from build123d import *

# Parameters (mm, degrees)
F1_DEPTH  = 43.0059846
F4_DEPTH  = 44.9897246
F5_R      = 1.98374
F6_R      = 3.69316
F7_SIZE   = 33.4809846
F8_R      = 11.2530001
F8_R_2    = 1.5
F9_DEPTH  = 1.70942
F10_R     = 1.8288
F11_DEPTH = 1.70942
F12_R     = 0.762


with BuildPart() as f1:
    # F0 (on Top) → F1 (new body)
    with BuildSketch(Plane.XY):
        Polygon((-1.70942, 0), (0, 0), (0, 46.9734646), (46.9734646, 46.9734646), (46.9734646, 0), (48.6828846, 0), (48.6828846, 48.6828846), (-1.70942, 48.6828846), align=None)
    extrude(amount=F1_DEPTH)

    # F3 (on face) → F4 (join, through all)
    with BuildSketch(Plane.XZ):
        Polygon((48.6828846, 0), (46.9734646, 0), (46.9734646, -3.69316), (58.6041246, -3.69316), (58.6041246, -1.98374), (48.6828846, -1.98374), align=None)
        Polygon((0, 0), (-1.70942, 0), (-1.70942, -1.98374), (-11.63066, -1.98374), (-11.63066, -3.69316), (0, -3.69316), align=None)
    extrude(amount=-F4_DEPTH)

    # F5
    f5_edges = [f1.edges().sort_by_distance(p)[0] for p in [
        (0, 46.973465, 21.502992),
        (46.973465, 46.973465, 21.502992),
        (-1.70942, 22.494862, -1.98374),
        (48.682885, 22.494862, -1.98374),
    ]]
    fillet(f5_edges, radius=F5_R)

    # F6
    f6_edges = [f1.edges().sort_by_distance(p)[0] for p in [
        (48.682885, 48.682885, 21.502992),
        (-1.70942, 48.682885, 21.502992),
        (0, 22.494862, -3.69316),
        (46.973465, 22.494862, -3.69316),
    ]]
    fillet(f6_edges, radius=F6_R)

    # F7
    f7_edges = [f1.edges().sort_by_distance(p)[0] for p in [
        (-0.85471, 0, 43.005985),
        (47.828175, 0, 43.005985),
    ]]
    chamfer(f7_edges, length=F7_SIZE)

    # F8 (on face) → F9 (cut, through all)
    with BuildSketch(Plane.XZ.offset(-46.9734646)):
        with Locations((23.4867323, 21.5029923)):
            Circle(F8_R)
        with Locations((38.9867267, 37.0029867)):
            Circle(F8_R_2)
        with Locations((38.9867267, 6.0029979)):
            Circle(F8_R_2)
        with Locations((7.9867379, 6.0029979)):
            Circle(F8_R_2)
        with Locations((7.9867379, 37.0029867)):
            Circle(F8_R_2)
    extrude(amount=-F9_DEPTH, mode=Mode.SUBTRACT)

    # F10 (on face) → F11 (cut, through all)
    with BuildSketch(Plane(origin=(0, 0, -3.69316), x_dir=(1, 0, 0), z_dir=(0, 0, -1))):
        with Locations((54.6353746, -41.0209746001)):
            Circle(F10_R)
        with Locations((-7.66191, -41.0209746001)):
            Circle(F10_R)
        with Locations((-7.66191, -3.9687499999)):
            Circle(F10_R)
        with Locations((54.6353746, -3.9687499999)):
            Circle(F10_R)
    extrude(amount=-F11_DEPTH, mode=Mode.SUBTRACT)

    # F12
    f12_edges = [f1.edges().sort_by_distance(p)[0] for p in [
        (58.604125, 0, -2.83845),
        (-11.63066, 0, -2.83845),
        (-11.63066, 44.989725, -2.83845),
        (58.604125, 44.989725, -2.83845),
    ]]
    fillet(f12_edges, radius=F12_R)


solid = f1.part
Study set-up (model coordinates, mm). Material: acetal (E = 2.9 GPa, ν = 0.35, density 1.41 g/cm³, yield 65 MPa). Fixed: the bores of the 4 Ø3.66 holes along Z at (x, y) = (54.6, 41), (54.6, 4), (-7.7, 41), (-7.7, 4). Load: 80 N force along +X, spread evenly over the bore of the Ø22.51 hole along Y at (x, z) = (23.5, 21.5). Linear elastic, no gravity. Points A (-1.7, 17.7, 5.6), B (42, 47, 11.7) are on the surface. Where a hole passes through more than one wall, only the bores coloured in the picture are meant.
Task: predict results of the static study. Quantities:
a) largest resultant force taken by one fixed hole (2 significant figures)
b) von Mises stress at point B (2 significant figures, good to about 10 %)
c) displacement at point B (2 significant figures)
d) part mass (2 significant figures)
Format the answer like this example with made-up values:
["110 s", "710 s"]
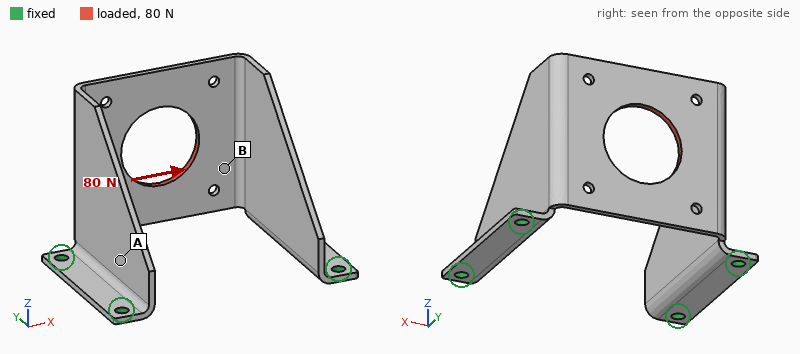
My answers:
["58 N", "4.8 MPa", "0.34 mm", "14 g"]
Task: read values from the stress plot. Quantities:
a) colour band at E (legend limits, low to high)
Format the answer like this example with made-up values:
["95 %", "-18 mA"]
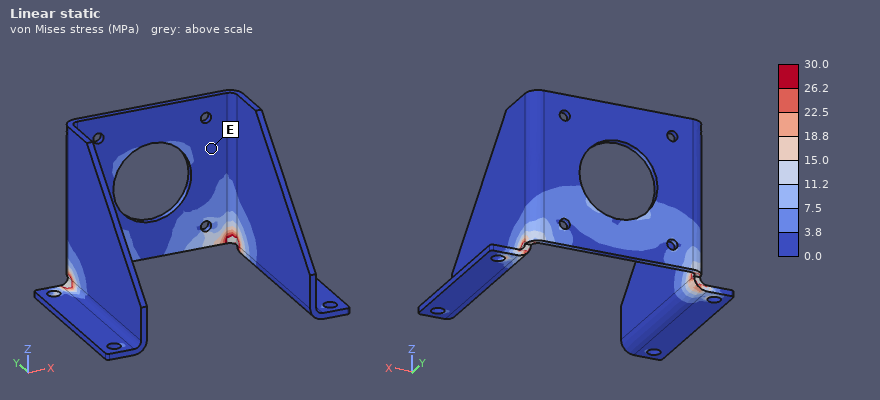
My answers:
["0.0 to 3.8 MPa"]
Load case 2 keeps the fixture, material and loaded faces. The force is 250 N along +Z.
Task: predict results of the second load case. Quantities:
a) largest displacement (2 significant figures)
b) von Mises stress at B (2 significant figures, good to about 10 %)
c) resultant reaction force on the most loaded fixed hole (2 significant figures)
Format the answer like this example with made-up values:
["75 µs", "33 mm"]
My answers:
["0.95 mm", "5.3 MPa", "150 N"]
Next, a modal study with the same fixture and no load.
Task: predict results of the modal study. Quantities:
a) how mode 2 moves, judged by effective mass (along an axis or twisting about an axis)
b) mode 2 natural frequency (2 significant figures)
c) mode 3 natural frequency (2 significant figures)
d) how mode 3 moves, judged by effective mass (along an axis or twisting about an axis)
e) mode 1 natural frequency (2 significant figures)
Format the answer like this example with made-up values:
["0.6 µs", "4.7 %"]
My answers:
["along X", "580 Hz", "800 Hz", "along Y", "490 Hz"]
